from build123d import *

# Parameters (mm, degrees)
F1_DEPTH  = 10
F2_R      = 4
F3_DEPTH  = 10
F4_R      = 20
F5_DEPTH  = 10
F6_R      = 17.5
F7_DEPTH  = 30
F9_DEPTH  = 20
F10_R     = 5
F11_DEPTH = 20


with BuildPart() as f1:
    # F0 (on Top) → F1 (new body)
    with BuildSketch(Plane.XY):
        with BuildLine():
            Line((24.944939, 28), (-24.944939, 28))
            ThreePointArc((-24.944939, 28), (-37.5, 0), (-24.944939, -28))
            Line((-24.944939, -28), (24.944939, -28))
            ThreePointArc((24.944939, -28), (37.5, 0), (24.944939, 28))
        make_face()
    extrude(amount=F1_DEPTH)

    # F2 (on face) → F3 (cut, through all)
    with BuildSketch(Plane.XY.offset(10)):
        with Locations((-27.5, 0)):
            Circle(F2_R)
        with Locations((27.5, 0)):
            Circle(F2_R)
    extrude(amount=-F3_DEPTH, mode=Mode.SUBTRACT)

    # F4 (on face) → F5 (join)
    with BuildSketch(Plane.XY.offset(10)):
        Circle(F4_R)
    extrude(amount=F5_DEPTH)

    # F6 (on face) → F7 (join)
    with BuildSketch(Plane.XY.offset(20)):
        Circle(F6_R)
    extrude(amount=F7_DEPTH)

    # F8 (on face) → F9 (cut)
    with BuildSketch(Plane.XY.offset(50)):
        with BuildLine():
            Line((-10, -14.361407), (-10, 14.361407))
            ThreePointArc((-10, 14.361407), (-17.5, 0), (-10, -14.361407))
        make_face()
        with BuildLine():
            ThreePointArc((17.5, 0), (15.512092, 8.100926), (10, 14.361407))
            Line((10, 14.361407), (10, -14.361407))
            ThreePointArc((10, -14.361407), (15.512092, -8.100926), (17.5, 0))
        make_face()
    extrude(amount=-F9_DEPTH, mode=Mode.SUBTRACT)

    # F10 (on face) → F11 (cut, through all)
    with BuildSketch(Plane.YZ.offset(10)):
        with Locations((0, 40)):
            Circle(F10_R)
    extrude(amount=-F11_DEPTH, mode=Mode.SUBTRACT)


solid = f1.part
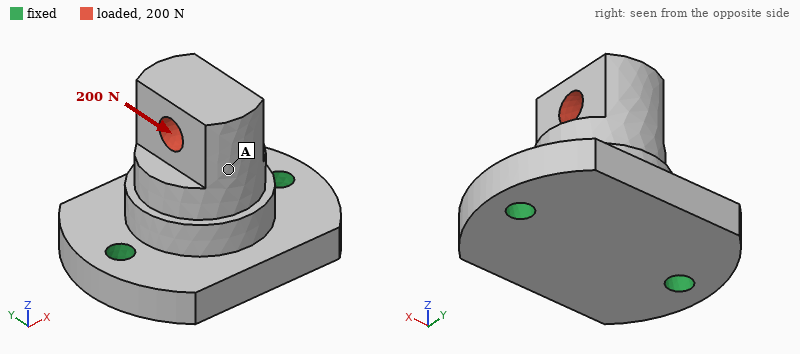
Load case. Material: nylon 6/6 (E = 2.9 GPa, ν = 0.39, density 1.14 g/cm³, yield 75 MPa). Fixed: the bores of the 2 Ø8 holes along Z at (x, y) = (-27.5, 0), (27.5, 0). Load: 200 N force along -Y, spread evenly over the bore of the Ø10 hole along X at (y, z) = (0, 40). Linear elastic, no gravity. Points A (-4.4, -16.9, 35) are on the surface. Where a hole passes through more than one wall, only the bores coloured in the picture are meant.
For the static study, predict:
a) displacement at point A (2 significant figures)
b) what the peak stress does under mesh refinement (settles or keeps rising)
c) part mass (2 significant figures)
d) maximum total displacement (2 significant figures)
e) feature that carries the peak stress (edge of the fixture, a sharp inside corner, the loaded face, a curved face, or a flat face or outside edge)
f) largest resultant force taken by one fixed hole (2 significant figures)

0.12 mm
keeps rising
80 g
0.18 mm
edge of the fixture
100 N
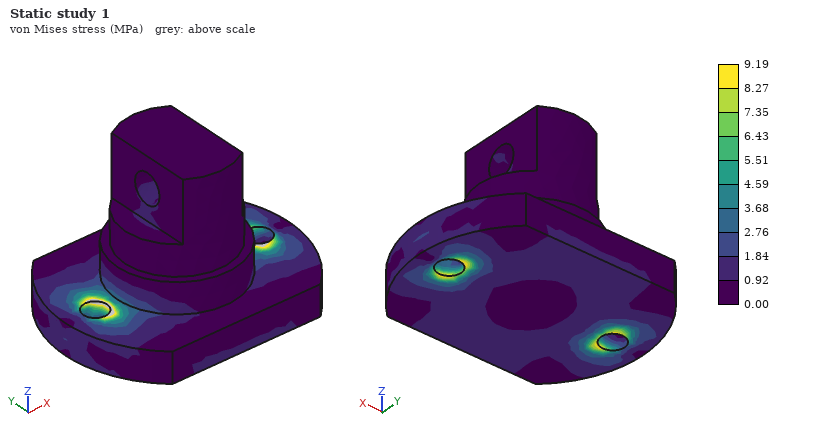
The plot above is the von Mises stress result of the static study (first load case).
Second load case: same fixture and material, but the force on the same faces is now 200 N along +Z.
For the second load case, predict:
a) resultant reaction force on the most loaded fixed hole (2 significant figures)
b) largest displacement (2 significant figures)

110 N
13 µm
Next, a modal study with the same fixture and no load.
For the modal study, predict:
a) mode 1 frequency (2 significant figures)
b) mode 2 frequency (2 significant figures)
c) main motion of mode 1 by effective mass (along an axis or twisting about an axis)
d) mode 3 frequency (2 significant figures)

1200 Hz
3000 Hz
along Y
3100 Hz
